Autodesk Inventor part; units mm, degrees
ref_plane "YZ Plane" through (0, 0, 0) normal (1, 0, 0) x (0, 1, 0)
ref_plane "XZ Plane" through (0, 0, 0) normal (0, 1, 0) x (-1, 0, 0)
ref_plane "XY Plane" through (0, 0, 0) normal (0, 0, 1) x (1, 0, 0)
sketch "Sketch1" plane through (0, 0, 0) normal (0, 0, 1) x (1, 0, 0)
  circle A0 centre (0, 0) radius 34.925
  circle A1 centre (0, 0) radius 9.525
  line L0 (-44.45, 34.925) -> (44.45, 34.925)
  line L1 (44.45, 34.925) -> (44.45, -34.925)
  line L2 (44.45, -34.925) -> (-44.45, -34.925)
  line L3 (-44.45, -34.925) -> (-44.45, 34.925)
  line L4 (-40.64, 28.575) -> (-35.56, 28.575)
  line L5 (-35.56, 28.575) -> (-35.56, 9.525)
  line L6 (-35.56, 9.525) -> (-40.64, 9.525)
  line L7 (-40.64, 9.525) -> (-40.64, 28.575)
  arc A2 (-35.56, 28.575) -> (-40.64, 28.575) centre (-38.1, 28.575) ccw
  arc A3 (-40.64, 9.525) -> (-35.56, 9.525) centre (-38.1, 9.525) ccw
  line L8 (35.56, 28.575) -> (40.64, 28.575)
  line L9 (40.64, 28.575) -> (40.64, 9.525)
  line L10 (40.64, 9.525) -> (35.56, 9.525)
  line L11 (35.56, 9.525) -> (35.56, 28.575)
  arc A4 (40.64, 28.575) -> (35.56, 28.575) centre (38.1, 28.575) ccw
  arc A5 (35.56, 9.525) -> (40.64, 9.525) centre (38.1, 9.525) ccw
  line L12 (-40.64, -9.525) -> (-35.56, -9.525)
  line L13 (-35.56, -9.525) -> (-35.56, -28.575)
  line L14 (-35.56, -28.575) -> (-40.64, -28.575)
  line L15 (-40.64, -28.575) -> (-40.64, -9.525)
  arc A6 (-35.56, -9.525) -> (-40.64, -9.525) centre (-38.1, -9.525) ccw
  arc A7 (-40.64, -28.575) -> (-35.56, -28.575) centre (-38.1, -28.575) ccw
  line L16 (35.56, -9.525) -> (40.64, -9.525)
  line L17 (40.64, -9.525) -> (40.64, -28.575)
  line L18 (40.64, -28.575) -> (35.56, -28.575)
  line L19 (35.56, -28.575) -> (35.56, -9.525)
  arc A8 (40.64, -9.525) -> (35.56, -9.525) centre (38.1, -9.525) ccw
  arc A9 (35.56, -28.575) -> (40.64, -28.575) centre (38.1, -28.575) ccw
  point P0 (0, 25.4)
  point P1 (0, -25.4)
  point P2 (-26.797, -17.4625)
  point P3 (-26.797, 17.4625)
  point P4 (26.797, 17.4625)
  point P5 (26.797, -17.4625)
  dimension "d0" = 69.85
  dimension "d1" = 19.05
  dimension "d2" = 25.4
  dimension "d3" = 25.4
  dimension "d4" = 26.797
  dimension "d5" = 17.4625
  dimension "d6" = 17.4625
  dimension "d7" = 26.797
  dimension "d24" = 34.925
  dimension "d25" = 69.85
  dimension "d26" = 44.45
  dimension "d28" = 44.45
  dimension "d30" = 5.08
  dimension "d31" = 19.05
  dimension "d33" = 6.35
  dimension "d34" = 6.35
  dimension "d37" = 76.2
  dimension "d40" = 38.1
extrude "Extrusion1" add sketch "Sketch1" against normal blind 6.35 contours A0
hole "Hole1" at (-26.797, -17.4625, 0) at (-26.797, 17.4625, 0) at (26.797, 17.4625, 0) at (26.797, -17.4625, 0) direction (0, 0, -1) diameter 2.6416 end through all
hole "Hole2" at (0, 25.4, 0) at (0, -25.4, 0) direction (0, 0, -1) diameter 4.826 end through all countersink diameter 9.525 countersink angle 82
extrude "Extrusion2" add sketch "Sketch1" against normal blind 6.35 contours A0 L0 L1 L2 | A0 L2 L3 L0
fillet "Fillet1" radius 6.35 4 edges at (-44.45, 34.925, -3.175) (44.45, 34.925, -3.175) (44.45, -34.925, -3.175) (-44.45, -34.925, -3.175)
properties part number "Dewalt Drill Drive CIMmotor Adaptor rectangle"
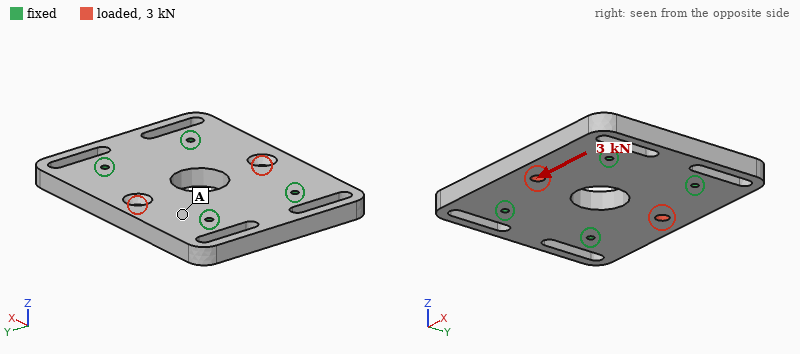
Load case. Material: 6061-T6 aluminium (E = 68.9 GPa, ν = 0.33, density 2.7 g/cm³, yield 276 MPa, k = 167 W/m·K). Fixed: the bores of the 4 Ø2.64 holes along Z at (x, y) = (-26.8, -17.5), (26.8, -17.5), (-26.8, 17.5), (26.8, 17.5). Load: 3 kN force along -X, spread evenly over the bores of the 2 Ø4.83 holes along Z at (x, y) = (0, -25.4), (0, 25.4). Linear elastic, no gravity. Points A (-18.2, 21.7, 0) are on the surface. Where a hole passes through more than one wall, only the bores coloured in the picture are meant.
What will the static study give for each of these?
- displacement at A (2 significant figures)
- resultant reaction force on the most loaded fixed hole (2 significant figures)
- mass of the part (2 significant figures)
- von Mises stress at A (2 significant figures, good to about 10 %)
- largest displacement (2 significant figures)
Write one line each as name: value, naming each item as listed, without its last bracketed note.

displacement at A: 1.7 µm
resultant reaction force on the most loaded fixed hole: 760 N
mass of the part: 92 g
von Mises stress at A: 6.8 MPa
largest displacement: 5.0 µm
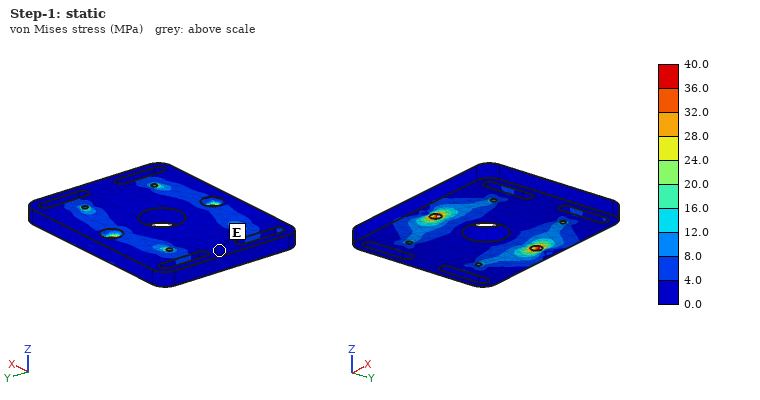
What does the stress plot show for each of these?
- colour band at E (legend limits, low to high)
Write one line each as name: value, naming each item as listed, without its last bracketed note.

colour band at E: 0.0 to 4.0 MPa
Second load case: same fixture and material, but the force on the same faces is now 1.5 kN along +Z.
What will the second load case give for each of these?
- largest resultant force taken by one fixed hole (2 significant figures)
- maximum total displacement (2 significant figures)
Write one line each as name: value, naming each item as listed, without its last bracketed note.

largest resultant force taken by one fixed hole: 380 N
maximum total displacement: 42 µm
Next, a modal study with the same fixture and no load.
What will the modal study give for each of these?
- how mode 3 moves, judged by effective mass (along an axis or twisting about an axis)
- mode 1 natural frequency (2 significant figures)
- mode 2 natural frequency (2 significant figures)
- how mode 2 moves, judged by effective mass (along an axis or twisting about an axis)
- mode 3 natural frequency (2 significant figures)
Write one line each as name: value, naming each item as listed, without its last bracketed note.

how mode 3 moves, judged by effective mass: along Z
mode 1 natural frequency: 7100 Hz
mode 2 natural frequency: 8000 Hz
how mode 2 moves, judged by effective mass: twisting about X
mode 3 natural frequency: 9500 Hz
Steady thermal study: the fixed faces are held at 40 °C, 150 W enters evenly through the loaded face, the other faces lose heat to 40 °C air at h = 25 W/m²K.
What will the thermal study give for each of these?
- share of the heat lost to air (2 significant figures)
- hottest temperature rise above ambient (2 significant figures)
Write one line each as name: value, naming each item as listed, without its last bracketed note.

share of the heat lost to air: 3.8 %
hottest temperature rise above ambient: 57 K
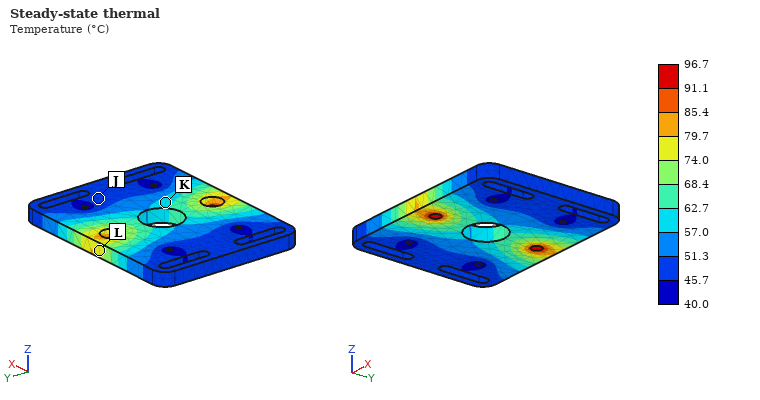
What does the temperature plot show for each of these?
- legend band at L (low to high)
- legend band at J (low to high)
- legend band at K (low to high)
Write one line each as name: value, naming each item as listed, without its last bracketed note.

legend band at L: 74.0 to 79.7 °C
legend band at J: 45.7 to 51.3 °C
legend band at K: 57.0 to 62.7 °C
